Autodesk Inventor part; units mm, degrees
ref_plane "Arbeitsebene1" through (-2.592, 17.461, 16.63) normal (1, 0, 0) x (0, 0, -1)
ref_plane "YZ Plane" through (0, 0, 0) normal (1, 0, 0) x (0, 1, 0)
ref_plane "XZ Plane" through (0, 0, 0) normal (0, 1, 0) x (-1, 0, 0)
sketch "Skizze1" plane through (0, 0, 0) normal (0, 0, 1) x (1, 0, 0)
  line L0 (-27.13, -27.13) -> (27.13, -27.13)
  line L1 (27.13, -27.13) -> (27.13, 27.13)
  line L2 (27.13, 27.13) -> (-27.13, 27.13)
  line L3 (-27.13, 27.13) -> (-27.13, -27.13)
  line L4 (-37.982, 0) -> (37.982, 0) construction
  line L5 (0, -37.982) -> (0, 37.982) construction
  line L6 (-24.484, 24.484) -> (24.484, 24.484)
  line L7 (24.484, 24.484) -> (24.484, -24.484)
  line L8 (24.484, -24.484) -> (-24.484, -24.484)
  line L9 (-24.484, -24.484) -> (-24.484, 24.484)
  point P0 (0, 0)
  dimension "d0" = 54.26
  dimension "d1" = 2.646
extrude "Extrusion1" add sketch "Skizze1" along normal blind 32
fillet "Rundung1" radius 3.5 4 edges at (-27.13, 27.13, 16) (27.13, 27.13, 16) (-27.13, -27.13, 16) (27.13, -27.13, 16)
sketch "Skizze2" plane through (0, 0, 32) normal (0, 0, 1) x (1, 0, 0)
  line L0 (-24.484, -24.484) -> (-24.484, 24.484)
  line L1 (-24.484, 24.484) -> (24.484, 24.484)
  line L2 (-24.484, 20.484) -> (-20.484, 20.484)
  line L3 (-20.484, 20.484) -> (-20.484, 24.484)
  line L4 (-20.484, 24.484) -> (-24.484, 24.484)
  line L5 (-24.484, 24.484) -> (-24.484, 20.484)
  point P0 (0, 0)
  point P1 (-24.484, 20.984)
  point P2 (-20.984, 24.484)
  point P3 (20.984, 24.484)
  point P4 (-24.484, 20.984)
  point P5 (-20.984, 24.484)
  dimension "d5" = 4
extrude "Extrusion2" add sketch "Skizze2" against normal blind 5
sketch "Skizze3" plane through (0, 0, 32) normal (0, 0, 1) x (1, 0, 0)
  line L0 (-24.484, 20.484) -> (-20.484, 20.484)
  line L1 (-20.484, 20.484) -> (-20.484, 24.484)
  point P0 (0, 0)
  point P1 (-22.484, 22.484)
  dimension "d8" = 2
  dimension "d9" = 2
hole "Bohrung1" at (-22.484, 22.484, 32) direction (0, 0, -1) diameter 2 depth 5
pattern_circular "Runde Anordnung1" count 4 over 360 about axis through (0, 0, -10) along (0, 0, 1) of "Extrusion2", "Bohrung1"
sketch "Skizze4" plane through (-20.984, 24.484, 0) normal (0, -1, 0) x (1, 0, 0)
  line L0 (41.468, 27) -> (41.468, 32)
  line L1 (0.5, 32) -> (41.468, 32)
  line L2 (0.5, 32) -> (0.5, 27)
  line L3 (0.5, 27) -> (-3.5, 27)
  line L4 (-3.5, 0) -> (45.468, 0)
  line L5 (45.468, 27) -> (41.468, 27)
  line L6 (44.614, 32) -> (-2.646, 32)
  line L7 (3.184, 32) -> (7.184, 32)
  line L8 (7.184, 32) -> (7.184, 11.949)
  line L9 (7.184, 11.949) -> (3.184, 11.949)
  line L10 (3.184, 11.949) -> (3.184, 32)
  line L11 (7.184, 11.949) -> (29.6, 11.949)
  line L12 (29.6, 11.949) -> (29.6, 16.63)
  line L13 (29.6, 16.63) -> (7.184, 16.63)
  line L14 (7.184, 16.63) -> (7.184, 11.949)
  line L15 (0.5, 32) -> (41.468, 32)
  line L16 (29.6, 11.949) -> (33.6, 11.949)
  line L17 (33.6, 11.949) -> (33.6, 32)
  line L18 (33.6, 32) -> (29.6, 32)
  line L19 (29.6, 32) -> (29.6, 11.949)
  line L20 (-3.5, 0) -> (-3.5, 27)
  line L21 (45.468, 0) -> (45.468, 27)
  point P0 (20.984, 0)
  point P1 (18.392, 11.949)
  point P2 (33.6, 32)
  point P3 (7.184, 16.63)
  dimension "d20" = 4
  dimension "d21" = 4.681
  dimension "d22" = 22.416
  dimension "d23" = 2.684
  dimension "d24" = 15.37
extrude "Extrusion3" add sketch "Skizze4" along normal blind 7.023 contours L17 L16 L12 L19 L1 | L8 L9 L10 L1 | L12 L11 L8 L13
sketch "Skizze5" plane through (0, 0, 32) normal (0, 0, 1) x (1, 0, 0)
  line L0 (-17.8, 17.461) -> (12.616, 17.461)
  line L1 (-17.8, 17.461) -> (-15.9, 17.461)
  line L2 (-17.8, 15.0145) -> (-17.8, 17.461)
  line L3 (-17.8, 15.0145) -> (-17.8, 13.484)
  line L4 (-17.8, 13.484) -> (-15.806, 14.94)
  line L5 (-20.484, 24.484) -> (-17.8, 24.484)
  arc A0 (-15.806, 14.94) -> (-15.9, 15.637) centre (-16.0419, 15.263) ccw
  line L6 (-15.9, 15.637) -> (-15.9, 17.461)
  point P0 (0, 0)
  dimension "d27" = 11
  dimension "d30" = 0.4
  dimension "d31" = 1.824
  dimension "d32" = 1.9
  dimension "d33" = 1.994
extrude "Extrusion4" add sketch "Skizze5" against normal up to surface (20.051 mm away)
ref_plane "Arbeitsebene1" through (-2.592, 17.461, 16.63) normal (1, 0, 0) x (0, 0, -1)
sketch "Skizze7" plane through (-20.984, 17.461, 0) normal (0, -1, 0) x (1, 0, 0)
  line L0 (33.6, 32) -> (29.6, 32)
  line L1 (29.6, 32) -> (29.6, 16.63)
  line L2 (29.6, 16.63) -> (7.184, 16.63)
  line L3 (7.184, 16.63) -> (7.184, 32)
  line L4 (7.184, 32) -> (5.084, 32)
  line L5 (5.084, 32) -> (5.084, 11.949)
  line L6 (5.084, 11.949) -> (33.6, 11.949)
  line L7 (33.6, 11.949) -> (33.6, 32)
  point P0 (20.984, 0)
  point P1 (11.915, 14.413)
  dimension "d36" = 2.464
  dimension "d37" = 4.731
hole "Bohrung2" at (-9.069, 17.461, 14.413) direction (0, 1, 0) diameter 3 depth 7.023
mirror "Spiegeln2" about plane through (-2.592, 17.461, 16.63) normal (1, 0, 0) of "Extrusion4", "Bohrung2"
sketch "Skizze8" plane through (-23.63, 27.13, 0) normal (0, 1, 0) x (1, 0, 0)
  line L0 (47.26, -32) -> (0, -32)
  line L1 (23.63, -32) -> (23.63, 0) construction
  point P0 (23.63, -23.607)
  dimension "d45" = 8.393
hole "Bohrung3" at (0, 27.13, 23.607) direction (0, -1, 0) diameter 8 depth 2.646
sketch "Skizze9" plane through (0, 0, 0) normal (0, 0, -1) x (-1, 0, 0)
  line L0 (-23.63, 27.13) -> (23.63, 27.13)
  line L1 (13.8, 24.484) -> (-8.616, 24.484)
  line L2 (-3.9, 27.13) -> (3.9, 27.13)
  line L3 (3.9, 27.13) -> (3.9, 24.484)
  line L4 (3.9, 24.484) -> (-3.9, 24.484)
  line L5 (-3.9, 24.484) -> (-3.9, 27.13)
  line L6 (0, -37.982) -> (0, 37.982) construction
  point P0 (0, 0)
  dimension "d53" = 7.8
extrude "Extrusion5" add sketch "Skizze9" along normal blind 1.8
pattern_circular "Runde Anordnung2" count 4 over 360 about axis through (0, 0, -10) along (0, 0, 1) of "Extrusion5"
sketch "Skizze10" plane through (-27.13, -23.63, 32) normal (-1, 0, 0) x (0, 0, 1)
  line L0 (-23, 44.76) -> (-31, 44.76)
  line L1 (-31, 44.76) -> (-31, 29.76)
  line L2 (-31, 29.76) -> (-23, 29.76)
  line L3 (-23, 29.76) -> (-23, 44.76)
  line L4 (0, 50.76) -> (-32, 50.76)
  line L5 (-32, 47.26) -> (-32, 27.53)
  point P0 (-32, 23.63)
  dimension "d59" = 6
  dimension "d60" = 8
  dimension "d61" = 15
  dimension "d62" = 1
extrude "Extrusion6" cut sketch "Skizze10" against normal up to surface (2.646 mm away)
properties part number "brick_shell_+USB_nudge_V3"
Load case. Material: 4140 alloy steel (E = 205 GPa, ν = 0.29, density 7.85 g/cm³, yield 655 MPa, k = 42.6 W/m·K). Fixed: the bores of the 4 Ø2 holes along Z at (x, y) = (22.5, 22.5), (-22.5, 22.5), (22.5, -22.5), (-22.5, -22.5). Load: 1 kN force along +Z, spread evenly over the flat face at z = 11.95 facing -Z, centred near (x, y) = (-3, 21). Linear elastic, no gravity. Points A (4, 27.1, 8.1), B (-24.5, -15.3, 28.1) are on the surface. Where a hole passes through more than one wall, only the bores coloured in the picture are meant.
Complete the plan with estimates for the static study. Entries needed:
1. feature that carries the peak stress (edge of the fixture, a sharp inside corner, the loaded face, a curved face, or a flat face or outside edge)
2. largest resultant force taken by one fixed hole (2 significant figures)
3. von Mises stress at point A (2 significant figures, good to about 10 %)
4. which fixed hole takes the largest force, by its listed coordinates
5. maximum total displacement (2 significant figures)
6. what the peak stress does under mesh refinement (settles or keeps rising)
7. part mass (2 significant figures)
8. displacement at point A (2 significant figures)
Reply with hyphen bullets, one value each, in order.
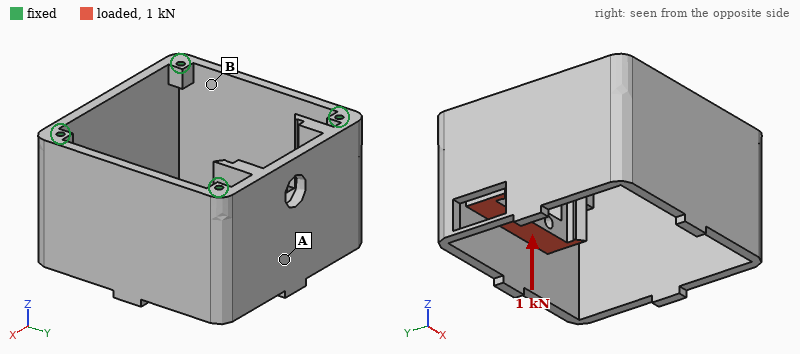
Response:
- edge of the fixture
- 540 N
- 17 MPa
- (-22.5, 22.5)
- 20 µm
- keeps rising
- 150 g
- 12 µm
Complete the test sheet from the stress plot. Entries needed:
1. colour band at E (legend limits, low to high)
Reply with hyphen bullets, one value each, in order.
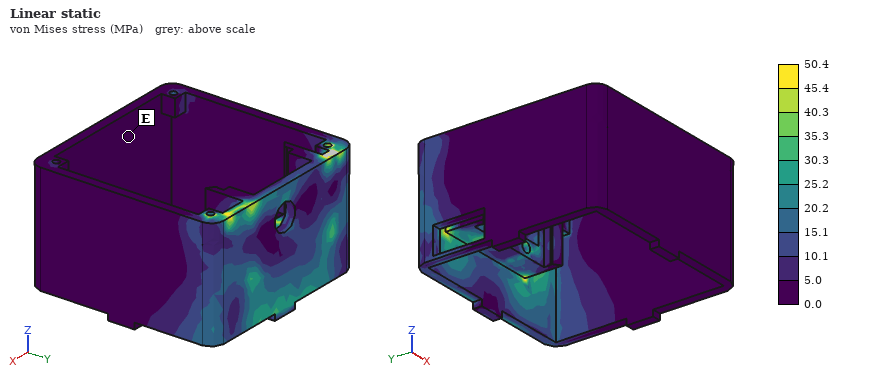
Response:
- 0.0 to 5.0 MPa
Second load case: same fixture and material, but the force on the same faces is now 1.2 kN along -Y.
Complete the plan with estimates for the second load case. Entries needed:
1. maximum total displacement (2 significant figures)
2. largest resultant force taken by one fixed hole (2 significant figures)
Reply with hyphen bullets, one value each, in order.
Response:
- 76 µm
- 490 N
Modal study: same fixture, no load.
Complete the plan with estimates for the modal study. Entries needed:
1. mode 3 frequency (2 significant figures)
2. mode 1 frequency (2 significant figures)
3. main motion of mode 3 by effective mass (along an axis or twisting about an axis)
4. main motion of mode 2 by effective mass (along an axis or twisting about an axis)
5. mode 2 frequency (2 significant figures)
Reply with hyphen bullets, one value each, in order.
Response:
- 4600 Hz
- 3500 Hz
- along Y
- along X
- 4400 Hz
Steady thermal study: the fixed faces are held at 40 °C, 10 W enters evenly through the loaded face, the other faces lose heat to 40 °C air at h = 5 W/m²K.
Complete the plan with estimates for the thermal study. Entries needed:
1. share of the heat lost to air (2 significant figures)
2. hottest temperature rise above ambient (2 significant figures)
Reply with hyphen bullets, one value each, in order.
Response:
- 9.5 %
- 44 K
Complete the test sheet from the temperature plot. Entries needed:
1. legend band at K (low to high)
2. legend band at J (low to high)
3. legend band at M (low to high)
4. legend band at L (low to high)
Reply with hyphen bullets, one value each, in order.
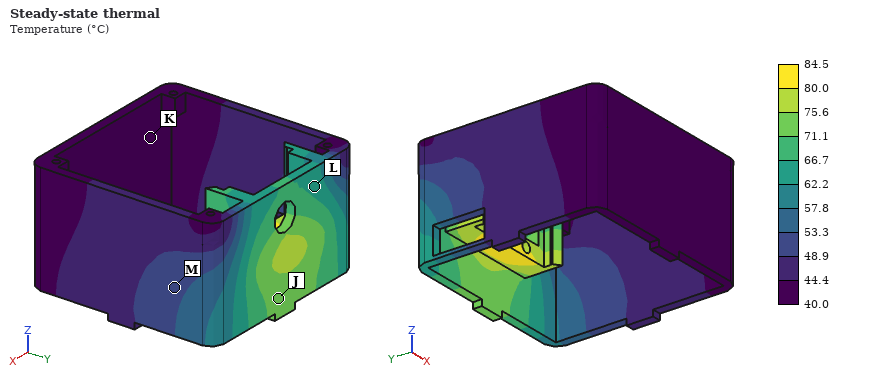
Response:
- 40.0 to 44.4 °C
- 71.1 to 75.6 °C
- 48.9 to 53.3 °C
- 62.2 to 66.7 °C
